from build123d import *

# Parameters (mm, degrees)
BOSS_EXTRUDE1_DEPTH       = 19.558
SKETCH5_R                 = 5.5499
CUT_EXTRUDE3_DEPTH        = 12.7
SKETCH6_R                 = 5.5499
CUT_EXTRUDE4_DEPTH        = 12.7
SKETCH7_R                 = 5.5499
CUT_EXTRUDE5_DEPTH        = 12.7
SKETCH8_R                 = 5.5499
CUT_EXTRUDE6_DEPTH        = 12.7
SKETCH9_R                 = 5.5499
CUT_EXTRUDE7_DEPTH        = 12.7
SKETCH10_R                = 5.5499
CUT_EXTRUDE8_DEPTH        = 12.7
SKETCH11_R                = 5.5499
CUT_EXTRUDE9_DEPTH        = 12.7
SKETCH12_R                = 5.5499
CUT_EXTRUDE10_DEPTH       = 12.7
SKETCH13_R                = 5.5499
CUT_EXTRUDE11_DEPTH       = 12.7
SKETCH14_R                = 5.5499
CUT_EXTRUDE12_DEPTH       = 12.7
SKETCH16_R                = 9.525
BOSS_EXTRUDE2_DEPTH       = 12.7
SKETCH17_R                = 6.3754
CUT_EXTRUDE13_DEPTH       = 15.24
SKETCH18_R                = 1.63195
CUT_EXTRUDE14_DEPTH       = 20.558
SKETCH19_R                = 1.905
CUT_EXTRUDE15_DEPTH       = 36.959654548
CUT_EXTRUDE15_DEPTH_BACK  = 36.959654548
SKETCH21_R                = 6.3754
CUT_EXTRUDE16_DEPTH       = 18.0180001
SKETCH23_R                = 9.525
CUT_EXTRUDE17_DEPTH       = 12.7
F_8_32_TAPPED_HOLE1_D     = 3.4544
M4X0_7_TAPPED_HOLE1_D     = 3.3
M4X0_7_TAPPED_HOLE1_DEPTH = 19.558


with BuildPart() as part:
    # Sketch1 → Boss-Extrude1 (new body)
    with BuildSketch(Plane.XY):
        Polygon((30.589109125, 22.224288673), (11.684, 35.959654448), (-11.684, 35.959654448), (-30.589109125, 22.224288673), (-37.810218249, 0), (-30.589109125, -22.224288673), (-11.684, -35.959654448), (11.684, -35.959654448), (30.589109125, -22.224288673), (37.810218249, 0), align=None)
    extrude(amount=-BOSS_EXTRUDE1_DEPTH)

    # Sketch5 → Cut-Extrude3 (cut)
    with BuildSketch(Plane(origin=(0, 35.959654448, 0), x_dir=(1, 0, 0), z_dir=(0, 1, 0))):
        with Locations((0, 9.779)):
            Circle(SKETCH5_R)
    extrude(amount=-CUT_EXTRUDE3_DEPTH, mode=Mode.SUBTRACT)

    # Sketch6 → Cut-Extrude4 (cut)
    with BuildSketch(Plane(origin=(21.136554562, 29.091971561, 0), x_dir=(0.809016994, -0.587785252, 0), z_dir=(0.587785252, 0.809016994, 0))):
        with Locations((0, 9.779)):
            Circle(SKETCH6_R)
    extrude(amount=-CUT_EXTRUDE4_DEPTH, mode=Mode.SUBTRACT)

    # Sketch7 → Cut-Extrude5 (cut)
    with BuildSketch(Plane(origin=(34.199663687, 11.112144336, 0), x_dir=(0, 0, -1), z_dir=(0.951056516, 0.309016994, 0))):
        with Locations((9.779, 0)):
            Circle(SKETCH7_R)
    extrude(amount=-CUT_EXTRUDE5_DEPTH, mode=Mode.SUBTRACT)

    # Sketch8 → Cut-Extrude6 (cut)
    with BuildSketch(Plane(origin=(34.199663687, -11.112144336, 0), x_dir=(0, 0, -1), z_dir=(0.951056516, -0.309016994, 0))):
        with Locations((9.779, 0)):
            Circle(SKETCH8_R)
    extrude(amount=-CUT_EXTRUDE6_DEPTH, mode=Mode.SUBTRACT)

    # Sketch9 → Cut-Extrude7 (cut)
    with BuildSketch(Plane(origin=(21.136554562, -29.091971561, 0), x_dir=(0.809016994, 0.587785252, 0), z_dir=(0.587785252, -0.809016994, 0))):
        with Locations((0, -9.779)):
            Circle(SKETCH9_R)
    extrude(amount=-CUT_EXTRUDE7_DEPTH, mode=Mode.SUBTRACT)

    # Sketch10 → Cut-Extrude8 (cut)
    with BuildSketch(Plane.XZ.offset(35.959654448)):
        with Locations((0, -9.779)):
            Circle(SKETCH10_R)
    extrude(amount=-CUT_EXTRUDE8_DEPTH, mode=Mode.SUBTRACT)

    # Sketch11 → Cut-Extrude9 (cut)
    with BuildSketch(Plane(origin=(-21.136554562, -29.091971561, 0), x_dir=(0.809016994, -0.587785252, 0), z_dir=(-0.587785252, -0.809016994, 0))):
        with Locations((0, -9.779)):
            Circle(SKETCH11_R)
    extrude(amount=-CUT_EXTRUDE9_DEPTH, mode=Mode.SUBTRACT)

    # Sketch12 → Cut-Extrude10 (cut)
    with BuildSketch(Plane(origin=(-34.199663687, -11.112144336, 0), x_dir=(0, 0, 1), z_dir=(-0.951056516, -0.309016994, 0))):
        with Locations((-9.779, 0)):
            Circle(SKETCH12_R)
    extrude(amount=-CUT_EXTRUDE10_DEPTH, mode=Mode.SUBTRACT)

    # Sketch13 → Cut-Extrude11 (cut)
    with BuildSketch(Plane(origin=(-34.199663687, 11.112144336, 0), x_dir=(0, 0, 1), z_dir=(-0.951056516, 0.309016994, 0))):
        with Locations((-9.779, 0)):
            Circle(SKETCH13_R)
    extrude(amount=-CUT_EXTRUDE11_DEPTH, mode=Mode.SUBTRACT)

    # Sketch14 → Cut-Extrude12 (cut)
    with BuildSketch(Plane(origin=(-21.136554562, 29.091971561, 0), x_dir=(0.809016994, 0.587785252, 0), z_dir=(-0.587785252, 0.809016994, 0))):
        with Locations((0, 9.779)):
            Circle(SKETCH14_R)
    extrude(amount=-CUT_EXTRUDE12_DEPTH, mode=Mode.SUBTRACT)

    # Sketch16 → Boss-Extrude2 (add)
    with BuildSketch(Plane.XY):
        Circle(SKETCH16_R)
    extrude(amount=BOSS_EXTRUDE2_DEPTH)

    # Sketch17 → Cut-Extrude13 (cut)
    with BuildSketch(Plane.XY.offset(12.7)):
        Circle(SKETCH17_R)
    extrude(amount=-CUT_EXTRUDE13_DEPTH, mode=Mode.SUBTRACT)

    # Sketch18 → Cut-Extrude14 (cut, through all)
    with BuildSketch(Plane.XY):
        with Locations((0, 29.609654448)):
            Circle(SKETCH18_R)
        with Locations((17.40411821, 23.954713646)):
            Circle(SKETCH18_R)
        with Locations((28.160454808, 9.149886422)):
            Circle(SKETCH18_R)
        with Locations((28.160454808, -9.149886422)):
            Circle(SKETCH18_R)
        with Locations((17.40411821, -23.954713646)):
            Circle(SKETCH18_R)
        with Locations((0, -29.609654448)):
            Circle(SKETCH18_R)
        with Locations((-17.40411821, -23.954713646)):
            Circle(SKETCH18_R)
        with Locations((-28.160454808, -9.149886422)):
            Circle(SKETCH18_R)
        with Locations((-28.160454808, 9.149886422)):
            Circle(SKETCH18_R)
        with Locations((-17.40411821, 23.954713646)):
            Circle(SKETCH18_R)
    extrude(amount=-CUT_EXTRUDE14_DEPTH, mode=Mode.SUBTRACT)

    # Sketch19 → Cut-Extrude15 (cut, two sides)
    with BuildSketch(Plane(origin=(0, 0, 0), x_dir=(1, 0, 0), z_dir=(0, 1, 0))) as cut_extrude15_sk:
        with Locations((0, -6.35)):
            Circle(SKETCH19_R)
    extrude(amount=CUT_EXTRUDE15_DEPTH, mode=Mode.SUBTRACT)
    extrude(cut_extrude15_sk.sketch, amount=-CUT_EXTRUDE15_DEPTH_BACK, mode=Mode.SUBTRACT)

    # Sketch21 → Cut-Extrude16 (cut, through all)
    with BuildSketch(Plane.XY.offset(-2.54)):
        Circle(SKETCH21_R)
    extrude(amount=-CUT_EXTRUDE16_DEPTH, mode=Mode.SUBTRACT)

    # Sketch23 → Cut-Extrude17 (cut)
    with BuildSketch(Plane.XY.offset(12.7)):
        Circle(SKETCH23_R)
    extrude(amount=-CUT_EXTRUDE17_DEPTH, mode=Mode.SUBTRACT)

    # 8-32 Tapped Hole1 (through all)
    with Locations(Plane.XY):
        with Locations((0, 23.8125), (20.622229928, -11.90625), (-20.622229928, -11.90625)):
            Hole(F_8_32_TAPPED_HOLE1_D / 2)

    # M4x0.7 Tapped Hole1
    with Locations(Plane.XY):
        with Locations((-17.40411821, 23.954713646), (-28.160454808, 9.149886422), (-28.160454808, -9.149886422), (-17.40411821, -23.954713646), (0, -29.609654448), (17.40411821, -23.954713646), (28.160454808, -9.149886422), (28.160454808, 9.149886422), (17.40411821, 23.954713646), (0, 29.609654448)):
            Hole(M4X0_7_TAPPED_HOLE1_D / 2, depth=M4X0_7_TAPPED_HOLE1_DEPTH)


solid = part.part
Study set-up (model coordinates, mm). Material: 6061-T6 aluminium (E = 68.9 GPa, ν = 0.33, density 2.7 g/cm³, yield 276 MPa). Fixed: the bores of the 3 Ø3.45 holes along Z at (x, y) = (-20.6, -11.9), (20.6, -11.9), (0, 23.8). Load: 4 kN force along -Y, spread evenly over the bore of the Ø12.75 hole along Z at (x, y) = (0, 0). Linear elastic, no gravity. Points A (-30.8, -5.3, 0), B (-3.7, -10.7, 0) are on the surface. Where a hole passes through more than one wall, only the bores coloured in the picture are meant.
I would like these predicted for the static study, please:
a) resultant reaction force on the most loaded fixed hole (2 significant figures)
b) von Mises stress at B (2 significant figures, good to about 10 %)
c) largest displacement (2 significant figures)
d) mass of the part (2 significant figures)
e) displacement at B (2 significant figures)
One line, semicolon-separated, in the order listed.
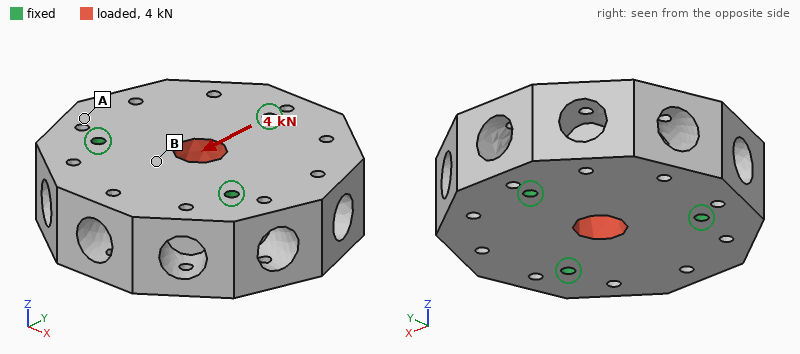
1.4 kN; 4.1 MPa; 2.3 µm; 180 g; 1.9 µm
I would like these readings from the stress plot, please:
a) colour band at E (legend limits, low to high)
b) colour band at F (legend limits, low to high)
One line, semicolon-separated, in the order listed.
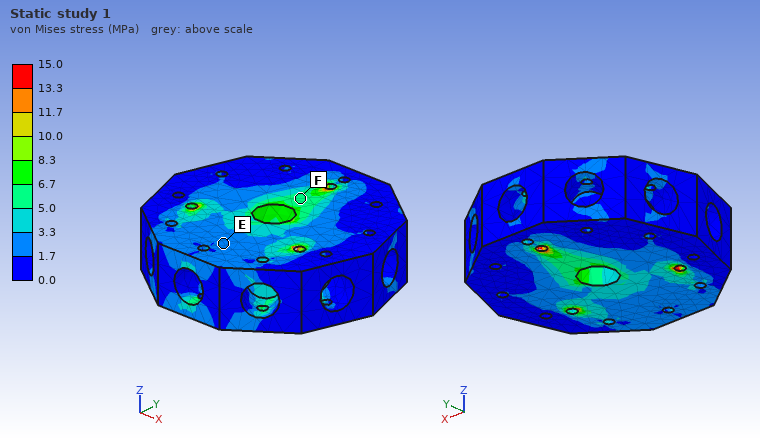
1.7 to 3.3 MPa; 5.0 to 6.7 MPa
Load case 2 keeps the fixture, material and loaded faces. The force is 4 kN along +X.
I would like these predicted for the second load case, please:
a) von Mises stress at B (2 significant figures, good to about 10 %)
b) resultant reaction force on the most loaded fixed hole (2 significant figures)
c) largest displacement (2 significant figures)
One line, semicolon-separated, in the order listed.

4.0 MPa; 1.4 kN; 2.2 µm
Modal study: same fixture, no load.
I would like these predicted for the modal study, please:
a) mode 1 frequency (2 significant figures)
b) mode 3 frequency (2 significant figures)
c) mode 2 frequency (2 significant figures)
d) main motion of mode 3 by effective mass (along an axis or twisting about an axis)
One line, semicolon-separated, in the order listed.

14 kHz; 17 kHz; 14 kHz; along Z
